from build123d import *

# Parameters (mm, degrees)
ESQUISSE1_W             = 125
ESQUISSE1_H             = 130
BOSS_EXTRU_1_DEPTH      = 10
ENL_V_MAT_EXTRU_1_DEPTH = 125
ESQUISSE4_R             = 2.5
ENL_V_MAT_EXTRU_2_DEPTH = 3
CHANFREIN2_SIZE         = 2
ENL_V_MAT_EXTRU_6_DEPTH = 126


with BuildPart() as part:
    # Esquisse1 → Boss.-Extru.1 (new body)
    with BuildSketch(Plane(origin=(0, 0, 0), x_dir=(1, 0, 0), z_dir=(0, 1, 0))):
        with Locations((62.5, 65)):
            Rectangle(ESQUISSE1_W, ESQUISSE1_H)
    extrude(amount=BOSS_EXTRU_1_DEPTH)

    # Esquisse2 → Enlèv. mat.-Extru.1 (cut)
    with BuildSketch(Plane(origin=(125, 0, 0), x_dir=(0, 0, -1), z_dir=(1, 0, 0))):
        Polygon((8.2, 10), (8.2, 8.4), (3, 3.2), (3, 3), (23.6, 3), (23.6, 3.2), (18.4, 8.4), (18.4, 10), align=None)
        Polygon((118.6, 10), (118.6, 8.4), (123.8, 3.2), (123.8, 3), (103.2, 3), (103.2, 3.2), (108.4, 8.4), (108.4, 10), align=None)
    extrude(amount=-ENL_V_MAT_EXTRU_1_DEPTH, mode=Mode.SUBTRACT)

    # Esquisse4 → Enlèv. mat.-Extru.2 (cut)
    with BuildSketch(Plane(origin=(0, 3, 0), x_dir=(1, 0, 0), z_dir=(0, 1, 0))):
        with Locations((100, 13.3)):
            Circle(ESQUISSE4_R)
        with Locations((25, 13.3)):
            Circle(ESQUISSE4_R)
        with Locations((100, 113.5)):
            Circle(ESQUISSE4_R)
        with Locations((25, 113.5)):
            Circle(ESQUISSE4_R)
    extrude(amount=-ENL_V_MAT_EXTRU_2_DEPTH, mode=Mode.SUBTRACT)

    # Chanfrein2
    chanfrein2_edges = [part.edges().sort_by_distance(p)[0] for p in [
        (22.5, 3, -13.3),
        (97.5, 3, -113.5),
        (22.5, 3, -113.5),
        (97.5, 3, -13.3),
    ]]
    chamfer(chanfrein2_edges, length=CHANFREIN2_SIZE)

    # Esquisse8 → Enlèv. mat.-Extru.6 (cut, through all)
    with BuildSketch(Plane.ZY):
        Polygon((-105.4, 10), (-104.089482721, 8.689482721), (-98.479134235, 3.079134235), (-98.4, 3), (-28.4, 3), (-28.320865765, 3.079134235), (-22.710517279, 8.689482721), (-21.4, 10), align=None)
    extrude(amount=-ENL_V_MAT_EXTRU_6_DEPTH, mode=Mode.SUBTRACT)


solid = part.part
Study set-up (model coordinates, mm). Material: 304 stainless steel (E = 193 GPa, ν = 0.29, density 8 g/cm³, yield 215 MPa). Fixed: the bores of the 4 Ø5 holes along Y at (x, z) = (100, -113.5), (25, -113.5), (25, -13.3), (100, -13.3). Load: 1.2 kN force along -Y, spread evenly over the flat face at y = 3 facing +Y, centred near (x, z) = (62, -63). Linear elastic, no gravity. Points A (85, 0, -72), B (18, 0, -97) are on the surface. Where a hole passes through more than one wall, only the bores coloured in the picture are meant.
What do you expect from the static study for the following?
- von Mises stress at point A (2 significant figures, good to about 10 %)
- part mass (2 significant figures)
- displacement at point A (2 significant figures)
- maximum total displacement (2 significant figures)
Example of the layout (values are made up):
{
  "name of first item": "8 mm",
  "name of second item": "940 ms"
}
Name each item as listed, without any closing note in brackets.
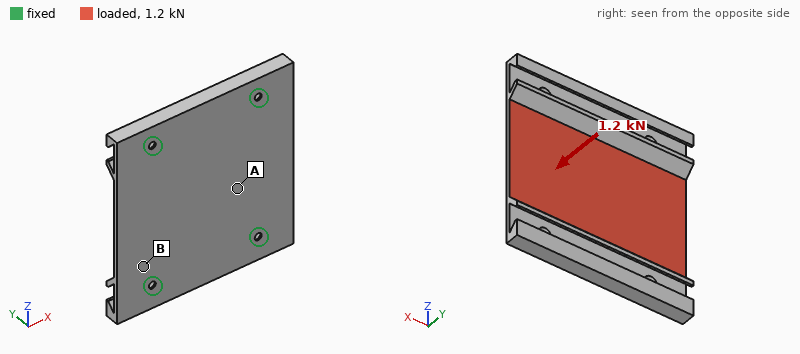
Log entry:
{
  "von Mises stress at point A": "37 MPa",
  "part mass": "560 g",
  "displacement at point A": "0.13 mm",
  "maximum total displacement": "0.14 mm"
}
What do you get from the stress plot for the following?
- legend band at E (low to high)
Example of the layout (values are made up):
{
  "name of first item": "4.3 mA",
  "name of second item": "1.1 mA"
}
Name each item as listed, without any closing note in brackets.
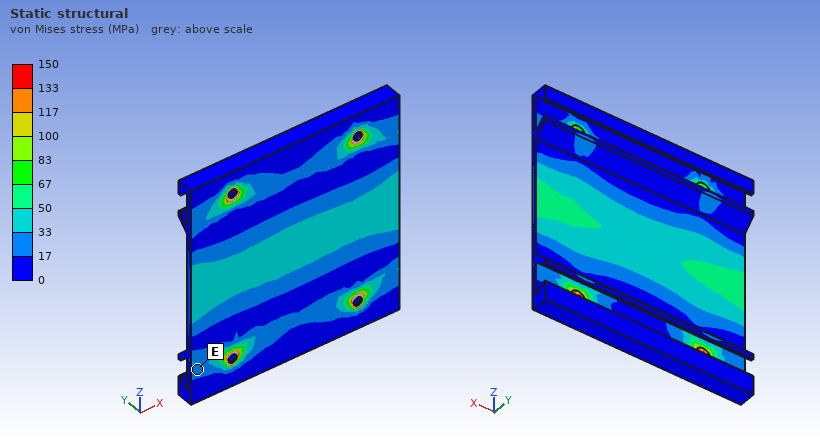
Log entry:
{
  "legend band at E": "17 to 33 MPa"
}
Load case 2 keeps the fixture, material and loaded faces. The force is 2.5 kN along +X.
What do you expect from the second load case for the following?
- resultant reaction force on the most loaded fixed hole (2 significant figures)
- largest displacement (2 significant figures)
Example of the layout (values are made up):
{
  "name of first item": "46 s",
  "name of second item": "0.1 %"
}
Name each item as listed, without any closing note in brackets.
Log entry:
{
  "resultant reaction force on the most loaded fixed hole": "650 N",
  "largest displacement": "13 µm"
}
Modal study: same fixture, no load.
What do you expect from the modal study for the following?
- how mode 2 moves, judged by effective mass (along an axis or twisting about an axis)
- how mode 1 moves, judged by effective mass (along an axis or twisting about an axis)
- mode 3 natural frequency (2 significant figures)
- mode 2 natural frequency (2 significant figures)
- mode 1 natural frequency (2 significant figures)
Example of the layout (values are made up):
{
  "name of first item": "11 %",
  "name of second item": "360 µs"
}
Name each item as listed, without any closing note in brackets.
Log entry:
{
  "how mode 2 moves, judged by effective mass": "twisting about Z",
  "how mode 1 moves, judged by effective mass": "along Y",
  "mode 3 natural frequency": "2400 Hz",
  "mode 2 natural frequency": "1500 Hz",
  "mode 1 natural frequency": "1100 Hz"
}
